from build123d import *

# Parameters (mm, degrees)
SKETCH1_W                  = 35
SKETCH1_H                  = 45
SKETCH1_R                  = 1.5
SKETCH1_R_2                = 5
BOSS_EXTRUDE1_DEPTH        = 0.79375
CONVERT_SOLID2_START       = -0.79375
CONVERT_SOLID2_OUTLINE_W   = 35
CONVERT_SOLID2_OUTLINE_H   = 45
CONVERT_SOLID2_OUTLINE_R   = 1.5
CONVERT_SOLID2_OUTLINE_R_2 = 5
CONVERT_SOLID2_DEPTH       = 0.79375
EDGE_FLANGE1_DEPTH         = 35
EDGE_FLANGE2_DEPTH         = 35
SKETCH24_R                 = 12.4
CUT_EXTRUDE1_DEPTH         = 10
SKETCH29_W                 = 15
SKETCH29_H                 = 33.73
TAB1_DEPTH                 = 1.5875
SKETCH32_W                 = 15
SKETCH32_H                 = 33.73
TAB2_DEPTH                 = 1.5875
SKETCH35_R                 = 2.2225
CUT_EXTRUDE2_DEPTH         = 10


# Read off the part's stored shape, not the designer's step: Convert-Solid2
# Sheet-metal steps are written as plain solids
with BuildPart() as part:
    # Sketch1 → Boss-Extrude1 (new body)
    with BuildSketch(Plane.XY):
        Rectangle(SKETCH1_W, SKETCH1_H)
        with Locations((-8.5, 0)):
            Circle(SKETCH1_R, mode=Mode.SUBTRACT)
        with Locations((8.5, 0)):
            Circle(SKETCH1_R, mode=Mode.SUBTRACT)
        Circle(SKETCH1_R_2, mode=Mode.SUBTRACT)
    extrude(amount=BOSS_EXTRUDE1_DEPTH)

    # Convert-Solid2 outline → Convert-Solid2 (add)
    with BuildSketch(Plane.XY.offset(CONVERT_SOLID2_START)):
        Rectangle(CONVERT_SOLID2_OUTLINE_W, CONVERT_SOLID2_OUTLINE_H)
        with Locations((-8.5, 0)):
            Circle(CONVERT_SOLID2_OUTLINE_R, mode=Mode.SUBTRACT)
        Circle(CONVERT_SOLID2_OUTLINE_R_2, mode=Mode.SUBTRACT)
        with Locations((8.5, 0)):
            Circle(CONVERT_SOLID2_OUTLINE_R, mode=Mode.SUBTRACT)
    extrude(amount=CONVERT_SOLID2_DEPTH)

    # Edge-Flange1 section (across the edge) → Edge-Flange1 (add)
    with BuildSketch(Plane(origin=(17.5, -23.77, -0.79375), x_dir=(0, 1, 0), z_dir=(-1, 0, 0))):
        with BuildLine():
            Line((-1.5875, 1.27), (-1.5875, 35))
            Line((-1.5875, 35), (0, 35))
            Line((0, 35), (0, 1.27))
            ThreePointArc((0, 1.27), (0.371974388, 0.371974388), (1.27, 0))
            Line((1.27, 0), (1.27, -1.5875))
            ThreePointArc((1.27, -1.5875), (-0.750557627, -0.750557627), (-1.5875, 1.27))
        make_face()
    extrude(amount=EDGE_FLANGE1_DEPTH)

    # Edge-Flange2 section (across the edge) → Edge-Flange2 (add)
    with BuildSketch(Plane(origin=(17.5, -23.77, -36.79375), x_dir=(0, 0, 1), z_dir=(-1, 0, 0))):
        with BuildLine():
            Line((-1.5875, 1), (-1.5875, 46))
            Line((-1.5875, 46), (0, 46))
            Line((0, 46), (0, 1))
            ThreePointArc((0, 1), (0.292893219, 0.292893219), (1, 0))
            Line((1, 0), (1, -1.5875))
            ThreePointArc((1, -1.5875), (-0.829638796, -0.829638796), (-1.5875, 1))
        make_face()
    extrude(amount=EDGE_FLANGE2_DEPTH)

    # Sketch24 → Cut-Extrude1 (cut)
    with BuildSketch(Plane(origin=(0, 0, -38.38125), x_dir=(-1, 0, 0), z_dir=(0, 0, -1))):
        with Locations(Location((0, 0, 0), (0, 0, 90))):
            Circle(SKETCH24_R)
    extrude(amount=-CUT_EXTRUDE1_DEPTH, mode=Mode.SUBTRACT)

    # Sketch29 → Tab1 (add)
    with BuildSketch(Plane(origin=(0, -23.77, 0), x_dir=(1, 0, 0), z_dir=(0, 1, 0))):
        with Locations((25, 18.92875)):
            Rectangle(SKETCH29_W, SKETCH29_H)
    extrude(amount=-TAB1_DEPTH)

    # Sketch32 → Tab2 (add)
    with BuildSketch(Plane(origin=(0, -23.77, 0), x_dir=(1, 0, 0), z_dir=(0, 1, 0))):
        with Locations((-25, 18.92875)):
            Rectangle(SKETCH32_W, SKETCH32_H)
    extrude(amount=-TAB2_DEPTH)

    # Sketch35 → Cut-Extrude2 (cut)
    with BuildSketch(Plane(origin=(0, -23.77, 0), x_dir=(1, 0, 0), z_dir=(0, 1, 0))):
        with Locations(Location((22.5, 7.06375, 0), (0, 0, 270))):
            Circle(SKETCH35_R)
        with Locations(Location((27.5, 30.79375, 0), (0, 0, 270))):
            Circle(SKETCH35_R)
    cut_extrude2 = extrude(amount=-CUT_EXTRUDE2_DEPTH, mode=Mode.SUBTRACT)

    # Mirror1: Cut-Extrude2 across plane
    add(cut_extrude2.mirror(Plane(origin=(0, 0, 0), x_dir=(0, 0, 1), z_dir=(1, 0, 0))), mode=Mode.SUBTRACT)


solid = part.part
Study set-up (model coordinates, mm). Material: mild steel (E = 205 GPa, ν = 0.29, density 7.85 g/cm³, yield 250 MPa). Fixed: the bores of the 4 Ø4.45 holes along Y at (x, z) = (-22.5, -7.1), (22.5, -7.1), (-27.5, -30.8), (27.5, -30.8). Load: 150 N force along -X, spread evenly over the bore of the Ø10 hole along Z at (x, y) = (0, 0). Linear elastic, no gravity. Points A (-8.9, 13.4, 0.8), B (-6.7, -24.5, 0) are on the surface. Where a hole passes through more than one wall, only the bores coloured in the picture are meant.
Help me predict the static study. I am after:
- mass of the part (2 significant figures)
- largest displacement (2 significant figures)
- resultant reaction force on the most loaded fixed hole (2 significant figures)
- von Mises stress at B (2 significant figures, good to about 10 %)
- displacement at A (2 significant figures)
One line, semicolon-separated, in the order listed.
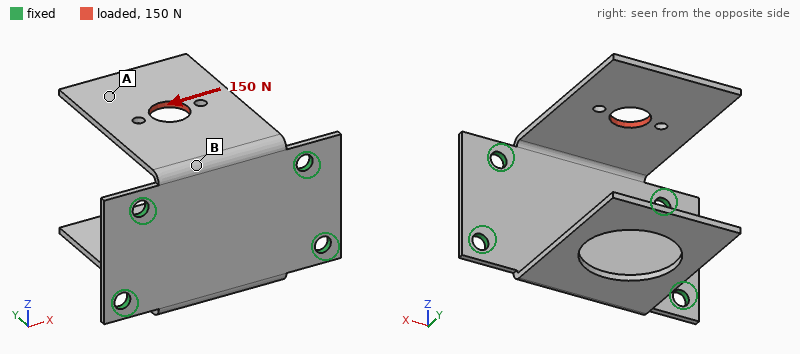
61 g; 60 µm; 130 N; 22 MPa; 43 µm
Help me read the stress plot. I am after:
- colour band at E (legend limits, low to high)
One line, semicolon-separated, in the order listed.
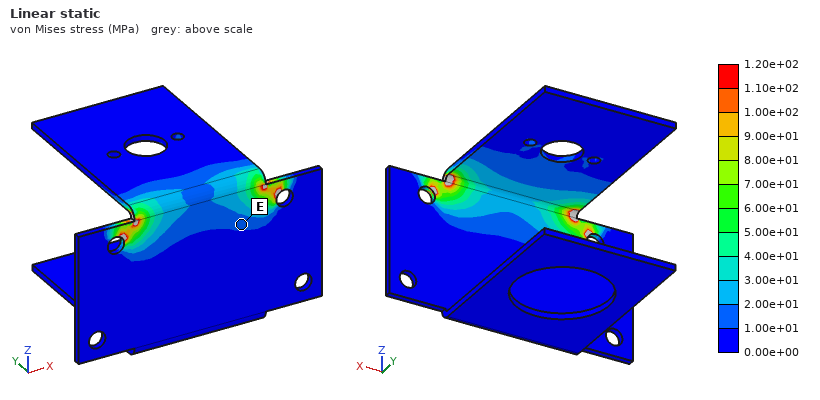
1.00e+01 to 2.00e+01 MPa
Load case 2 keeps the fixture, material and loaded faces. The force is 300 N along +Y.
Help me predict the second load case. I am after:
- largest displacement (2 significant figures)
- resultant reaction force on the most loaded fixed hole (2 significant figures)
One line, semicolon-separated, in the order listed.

0.19 mm; 180 N
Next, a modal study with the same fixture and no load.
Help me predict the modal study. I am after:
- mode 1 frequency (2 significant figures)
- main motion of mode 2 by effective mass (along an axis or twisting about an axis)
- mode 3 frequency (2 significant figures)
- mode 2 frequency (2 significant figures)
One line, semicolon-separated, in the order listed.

440 Hz; along Z; 1400 Hz; 470 Hz
